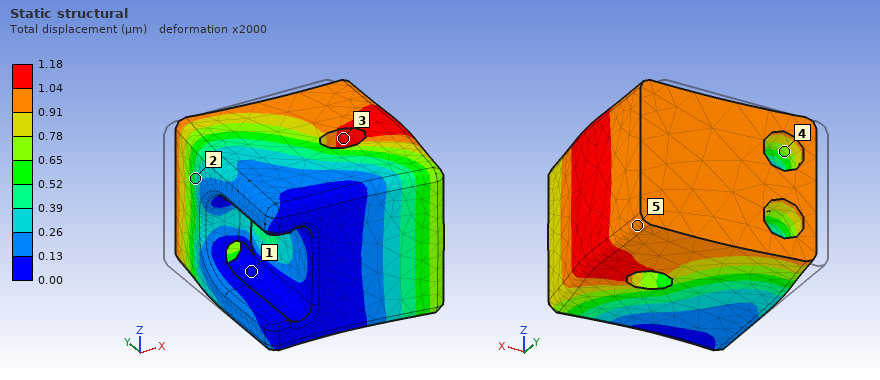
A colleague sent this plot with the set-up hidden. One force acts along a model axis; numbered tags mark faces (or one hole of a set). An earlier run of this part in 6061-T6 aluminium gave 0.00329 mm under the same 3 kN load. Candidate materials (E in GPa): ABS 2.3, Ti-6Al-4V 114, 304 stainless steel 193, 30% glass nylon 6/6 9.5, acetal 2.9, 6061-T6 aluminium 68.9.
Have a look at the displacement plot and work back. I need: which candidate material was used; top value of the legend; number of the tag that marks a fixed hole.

304 stainless steel
1.18 µm
1
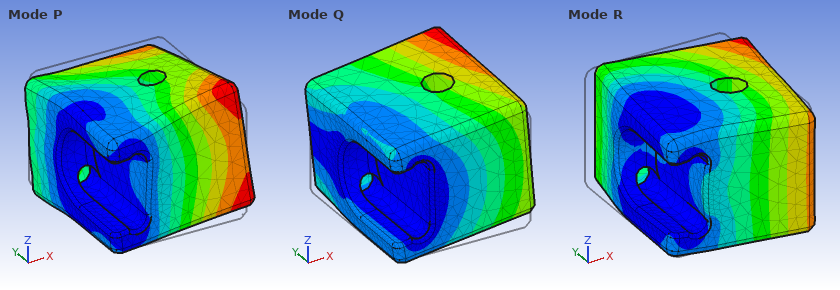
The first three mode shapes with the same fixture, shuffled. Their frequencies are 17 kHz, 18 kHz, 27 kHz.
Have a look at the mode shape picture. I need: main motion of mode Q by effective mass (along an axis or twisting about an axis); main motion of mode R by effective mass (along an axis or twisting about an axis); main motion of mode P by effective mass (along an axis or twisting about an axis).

along Z
along Y
twisting about X
